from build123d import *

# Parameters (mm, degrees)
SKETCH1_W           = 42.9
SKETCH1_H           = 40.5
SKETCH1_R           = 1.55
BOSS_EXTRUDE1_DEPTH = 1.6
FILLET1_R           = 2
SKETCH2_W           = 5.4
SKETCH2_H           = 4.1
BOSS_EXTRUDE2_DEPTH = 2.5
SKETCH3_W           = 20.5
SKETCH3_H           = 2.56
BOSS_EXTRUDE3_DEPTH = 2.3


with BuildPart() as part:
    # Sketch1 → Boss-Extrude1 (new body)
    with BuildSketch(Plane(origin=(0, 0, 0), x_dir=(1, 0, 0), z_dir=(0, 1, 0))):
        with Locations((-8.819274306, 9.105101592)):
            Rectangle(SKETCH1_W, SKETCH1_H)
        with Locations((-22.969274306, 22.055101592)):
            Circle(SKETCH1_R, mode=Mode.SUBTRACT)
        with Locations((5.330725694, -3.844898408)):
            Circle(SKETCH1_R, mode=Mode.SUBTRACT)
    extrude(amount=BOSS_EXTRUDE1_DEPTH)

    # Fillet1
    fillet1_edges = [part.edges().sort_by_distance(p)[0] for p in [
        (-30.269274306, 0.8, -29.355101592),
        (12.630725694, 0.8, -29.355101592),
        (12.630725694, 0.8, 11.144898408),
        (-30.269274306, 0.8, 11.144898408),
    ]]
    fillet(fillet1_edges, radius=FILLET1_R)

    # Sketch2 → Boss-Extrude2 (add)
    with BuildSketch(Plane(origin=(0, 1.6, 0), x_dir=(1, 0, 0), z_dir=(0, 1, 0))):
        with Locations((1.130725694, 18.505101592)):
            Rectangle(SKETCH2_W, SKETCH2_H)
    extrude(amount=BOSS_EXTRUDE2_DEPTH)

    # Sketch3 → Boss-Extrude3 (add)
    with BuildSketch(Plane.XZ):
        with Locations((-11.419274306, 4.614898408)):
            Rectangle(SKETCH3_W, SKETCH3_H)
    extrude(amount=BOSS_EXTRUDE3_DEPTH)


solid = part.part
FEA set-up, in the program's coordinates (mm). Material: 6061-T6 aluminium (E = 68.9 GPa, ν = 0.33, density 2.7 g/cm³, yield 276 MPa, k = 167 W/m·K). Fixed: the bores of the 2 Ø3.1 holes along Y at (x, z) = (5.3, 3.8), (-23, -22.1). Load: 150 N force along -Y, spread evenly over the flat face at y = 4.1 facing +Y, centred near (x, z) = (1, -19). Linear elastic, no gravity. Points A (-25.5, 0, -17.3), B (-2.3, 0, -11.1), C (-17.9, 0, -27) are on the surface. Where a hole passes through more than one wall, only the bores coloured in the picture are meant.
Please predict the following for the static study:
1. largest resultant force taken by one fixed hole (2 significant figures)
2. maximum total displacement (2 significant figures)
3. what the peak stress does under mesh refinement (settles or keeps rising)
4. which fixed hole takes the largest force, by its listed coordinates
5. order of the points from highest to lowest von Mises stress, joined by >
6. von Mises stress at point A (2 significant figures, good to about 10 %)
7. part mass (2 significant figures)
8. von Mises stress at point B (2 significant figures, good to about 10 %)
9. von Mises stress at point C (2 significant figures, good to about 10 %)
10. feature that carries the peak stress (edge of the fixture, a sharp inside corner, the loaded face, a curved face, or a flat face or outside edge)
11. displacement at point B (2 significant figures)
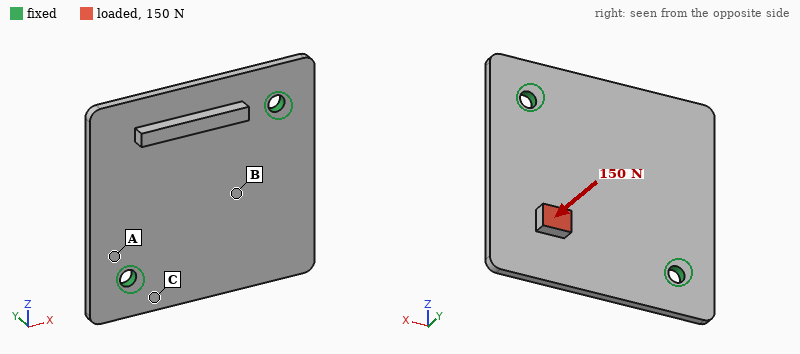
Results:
80 N
0.62 mm
keeps rising
(5.3, 3.8)
C > B > A
24 MPa
7.9 g
62 MPa
100 MPa
edge of the fixture
0.14 mm
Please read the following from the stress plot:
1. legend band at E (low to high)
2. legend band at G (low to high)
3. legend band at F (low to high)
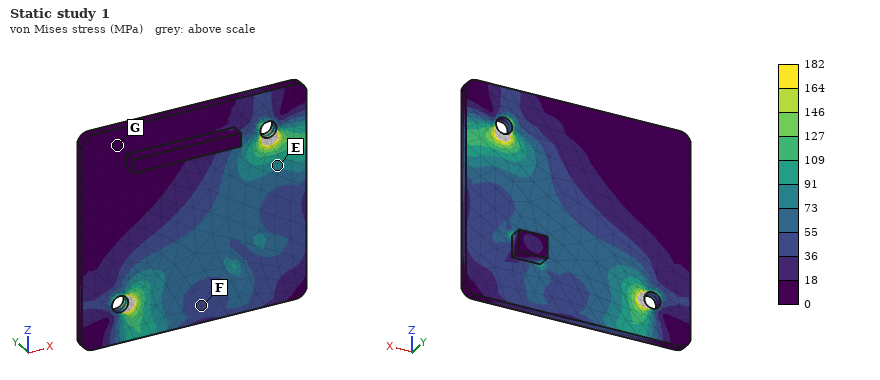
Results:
73 to 91 MPa
0 to 18 MPa
36 to 55 MPa
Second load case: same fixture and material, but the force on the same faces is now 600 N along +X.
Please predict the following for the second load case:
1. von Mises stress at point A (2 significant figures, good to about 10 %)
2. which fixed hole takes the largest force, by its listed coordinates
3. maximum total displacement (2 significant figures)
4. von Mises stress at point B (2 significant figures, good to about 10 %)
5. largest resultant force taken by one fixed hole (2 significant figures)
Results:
24 MPa
(-23, -22.1)
0.55 mm
85 MPa
430 N
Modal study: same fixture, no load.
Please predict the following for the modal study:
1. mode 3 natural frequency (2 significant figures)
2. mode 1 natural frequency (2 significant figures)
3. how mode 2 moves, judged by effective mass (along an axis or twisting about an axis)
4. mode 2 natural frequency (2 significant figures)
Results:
7100 Hz
1900 Hz
along Y
2500 Hz
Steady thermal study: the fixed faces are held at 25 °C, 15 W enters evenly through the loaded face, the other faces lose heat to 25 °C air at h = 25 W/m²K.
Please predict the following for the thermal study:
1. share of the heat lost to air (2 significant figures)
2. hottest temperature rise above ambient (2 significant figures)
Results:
9.0 %
50 K
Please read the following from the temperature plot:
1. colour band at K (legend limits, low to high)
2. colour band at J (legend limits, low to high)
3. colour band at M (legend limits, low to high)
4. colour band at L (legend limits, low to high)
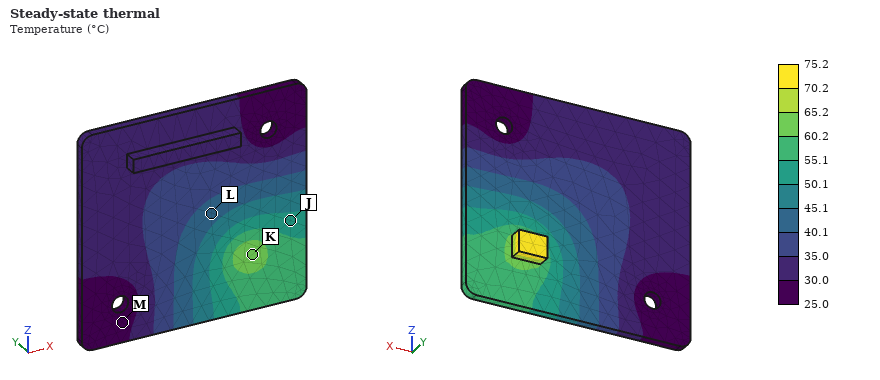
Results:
60.2 to 65.2 °C
50.1 to 55.1 °C
25.0 to 30.0 °C
40.1 to 45.1 °C
